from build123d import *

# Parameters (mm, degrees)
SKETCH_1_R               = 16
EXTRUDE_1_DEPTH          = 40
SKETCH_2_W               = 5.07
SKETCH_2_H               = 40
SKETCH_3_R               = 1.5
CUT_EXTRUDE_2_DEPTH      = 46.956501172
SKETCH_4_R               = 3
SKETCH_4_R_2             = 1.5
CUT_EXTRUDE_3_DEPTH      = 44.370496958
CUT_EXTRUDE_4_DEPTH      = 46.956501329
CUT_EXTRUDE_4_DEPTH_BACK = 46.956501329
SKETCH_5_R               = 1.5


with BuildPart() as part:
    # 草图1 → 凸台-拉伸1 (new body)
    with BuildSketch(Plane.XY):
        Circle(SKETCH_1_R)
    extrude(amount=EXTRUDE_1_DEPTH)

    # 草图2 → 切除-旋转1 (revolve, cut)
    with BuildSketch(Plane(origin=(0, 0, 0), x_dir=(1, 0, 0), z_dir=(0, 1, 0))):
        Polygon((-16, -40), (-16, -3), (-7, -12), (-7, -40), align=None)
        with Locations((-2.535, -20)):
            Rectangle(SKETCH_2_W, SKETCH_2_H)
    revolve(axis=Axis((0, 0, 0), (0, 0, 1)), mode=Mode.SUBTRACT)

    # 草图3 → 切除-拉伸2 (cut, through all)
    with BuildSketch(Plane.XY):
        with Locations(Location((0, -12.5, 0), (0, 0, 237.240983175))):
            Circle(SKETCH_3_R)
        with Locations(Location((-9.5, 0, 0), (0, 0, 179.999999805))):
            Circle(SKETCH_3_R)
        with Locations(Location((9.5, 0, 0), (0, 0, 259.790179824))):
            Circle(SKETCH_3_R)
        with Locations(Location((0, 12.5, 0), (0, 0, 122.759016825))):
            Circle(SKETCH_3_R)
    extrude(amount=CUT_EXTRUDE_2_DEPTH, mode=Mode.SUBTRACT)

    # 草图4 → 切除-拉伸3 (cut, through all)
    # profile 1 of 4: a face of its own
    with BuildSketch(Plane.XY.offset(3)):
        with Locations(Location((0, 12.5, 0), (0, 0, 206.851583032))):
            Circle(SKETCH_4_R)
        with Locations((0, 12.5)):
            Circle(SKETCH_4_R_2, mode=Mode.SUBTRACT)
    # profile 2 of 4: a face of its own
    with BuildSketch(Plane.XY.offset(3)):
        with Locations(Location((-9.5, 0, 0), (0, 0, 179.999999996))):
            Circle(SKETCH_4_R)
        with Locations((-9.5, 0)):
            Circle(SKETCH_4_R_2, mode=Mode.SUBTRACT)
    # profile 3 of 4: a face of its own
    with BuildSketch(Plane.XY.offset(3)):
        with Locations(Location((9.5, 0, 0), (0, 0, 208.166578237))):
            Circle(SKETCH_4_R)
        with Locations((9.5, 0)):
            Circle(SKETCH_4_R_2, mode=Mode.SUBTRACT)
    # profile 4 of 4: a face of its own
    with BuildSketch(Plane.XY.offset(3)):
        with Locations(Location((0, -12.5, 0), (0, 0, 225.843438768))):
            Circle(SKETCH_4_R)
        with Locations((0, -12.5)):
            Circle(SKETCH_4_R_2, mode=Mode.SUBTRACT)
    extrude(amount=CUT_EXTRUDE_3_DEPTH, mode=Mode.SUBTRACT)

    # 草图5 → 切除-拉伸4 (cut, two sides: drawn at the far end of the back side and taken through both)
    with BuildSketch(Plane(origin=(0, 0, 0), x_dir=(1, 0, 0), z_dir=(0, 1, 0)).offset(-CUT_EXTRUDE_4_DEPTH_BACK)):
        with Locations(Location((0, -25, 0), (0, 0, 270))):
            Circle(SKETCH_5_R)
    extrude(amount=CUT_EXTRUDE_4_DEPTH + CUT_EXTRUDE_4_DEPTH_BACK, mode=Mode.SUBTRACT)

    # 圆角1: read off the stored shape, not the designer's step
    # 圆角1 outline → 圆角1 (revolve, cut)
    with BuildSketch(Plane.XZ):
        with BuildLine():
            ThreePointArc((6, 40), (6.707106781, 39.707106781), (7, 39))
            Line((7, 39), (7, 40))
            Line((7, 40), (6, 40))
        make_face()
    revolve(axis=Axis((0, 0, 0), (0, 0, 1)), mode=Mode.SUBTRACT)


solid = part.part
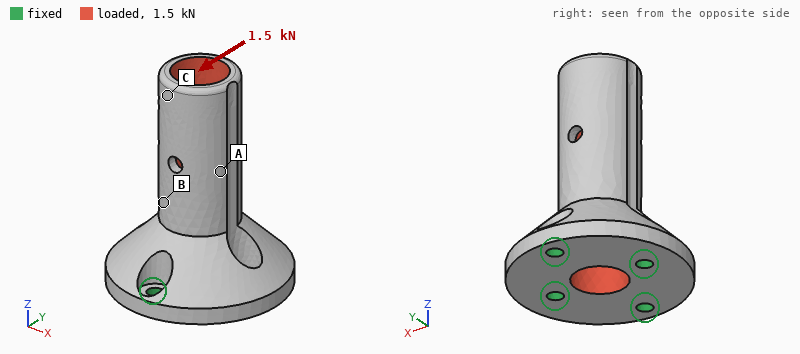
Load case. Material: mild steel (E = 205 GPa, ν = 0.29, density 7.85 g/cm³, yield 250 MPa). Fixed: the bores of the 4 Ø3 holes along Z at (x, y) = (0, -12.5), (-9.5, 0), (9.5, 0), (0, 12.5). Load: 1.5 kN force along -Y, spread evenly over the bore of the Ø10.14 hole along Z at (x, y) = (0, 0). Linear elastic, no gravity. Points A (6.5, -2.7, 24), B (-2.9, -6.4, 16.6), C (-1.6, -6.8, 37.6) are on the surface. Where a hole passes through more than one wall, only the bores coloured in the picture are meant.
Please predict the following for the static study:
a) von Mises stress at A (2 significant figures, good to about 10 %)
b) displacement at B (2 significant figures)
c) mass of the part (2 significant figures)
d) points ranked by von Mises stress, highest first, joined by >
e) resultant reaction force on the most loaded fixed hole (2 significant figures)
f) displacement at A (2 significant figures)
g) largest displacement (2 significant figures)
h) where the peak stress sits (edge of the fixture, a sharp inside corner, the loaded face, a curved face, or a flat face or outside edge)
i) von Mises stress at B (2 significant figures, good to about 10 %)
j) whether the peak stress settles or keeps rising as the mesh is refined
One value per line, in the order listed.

23 MPa
7.1 µm
53 g
B > A > C
1.2 kN
13 µm
28 µm
edge of the fixture
45 MPa
keeps rising
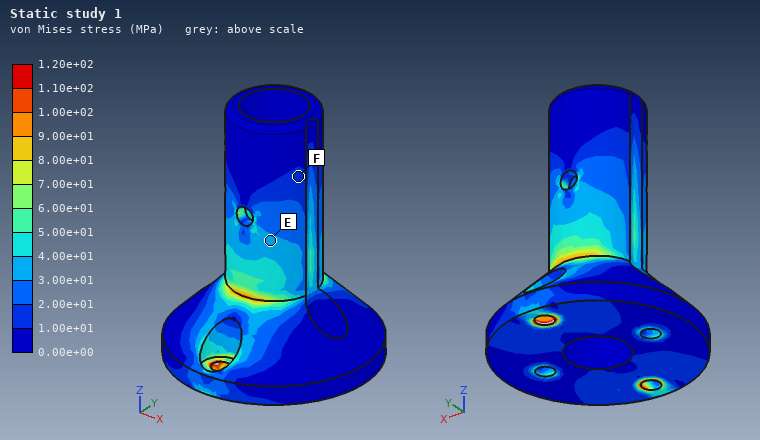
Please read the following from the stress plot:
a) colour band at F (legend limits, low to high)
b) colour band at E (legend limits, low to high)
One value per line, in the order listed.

1.00e+01 to 2.00e+01 MPa
3.00e+01 to 4.00e+01 MPa
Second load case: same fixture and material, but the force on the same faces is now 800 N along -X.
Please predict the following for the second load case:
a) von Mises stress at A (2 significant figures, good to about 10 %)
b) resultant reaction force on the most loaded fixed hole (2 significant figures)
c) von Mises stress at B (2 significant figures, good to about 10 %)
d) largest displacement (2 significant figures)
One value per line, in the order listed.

16 MPa
760 N
20 MPa
17 µm
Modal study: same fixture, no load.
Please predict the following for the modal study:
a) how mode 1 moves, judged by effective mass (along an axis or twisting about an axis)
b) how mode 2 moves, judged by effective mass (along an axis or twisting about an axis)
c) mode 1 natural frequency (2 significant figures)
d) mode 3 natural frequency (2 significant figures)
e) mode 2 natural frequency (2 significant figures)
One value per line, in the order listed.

along X
along Y
8900 Hz
25 kHz
9400 Hz
